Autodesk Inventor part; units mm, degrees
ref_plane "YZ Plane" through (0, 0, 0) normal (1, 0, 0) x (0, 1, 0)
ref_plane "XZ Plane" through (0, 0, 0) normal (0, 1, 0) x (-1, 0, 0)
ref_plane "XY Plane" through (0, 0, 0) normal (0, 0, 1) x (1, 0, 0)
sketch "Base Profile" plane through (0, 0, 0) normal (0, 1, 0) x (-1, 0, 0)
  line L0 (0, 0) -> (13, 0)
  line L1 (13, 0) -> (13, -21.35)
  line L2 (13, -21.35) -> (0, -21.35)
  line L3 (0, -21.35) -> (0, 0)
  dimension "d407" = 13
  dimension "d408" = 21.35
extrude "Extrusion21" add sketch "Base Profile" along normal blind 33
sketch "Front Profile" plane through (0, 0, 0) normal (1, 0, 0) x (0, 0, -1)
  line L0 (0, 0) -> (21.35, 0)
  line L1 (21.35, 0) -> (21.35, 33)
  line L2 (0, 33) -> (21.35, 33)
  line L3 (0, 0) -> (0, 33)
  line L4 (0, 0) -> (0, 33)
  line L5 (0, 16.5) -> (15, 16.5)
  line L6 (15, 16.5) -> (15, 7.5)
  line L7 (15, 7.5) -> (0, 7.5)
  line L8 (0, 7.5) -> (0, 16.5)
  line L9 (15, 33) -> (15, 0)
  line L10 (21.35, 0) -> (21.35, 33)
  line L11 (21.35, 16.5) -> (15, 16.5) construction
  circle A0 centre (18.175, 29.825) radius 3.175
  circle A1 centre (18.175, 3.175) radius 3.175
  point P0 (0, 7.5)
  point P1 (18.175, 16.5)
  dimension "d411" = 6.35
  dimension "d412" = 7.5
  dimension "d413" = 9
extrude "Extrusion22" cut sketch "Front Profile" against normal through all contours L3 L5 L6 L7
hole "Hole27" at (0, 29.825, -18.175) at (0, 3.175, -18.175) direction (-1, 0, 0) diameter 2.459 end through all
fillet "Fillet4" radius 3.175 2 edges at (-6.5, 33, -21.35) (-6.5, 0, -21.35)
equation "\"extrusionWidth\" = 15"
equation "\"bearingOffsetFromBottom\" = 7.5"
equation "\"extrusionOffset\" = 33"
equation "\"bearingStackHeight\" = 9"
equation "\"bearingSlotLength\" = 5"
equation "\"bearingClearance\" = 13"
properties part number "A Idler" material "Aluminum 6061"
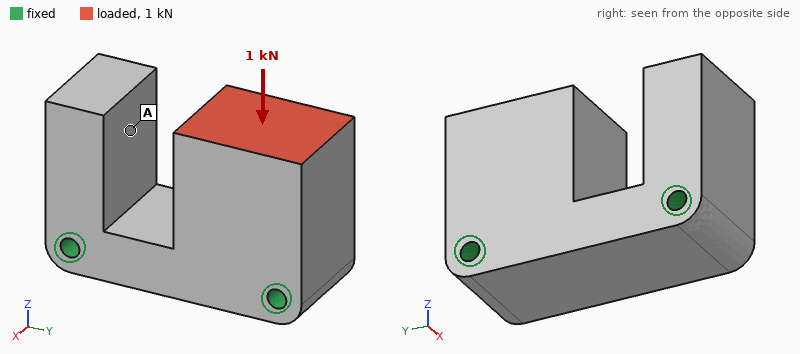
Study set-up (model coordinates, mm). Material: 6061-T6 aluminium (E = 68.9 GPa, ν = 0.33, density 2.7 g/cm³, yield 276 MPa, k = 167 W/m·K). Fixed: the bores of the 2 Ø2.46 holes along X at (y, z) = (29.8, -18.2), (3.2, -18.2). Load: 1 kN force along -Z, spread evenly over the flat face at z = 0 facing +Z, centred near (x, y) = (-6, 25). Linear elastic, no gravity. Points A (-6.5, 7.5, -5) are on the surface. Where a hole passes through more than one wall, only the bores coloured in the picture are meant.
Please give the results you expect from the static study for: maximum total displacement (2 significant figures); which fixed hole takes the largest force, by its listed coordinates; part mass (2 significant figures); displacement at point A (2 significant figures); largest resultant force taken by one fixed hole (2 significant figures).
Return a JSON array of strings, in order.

["6.6 µm", "(29.8, -18.2)", "20 g", "2.5 µm", "820 N"]
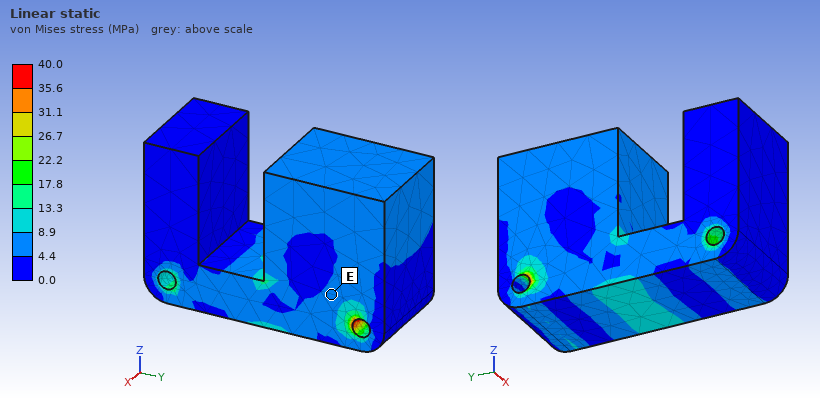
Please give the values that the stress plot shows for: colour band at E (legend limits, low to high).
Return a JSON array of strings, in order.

["4.4 to 8.9 MPa"]
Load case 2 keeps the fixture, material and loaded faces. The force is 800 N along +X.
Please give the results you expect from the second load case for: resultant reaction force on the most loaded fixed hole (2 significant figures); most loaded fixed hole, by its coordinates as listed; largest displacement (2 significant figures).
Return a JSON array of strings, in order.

["730 N", "(29.8, -18.2)", "21 µm"]
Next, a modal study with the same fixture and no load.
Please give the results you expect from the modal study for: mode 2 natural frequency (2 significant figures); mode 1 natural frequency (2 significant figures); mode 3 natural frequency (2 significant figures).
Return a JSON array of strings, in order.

["18 kHz", "13 kHz", "18 kHz"]
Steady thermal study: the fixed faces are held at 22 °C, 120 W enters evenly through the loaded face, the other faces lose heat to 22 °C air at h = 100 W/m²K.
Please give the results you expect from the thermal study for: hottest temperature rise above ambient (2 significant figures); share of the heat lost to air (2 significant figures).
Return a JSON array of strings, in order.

["69 K", "4.0 %"]
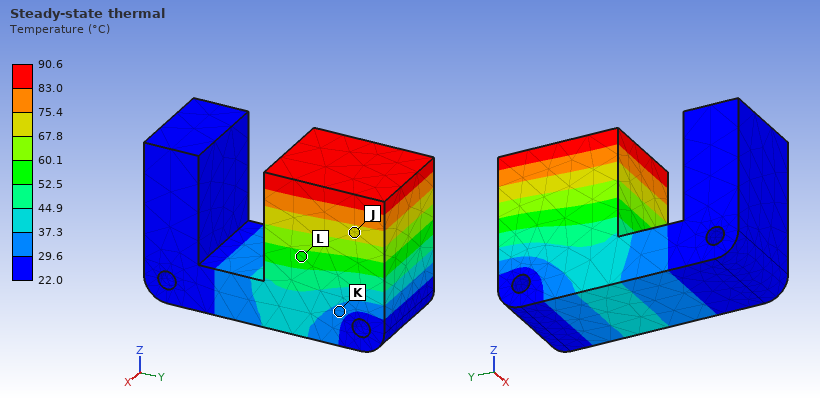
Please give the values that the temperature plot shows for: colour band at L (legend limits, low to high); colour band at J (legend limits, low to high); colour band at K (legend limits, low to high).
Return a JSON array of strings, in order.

["52.5 to 60.1 °C", "67.8 to 75.4 °C", "29.6 to 37.3 °C"]
